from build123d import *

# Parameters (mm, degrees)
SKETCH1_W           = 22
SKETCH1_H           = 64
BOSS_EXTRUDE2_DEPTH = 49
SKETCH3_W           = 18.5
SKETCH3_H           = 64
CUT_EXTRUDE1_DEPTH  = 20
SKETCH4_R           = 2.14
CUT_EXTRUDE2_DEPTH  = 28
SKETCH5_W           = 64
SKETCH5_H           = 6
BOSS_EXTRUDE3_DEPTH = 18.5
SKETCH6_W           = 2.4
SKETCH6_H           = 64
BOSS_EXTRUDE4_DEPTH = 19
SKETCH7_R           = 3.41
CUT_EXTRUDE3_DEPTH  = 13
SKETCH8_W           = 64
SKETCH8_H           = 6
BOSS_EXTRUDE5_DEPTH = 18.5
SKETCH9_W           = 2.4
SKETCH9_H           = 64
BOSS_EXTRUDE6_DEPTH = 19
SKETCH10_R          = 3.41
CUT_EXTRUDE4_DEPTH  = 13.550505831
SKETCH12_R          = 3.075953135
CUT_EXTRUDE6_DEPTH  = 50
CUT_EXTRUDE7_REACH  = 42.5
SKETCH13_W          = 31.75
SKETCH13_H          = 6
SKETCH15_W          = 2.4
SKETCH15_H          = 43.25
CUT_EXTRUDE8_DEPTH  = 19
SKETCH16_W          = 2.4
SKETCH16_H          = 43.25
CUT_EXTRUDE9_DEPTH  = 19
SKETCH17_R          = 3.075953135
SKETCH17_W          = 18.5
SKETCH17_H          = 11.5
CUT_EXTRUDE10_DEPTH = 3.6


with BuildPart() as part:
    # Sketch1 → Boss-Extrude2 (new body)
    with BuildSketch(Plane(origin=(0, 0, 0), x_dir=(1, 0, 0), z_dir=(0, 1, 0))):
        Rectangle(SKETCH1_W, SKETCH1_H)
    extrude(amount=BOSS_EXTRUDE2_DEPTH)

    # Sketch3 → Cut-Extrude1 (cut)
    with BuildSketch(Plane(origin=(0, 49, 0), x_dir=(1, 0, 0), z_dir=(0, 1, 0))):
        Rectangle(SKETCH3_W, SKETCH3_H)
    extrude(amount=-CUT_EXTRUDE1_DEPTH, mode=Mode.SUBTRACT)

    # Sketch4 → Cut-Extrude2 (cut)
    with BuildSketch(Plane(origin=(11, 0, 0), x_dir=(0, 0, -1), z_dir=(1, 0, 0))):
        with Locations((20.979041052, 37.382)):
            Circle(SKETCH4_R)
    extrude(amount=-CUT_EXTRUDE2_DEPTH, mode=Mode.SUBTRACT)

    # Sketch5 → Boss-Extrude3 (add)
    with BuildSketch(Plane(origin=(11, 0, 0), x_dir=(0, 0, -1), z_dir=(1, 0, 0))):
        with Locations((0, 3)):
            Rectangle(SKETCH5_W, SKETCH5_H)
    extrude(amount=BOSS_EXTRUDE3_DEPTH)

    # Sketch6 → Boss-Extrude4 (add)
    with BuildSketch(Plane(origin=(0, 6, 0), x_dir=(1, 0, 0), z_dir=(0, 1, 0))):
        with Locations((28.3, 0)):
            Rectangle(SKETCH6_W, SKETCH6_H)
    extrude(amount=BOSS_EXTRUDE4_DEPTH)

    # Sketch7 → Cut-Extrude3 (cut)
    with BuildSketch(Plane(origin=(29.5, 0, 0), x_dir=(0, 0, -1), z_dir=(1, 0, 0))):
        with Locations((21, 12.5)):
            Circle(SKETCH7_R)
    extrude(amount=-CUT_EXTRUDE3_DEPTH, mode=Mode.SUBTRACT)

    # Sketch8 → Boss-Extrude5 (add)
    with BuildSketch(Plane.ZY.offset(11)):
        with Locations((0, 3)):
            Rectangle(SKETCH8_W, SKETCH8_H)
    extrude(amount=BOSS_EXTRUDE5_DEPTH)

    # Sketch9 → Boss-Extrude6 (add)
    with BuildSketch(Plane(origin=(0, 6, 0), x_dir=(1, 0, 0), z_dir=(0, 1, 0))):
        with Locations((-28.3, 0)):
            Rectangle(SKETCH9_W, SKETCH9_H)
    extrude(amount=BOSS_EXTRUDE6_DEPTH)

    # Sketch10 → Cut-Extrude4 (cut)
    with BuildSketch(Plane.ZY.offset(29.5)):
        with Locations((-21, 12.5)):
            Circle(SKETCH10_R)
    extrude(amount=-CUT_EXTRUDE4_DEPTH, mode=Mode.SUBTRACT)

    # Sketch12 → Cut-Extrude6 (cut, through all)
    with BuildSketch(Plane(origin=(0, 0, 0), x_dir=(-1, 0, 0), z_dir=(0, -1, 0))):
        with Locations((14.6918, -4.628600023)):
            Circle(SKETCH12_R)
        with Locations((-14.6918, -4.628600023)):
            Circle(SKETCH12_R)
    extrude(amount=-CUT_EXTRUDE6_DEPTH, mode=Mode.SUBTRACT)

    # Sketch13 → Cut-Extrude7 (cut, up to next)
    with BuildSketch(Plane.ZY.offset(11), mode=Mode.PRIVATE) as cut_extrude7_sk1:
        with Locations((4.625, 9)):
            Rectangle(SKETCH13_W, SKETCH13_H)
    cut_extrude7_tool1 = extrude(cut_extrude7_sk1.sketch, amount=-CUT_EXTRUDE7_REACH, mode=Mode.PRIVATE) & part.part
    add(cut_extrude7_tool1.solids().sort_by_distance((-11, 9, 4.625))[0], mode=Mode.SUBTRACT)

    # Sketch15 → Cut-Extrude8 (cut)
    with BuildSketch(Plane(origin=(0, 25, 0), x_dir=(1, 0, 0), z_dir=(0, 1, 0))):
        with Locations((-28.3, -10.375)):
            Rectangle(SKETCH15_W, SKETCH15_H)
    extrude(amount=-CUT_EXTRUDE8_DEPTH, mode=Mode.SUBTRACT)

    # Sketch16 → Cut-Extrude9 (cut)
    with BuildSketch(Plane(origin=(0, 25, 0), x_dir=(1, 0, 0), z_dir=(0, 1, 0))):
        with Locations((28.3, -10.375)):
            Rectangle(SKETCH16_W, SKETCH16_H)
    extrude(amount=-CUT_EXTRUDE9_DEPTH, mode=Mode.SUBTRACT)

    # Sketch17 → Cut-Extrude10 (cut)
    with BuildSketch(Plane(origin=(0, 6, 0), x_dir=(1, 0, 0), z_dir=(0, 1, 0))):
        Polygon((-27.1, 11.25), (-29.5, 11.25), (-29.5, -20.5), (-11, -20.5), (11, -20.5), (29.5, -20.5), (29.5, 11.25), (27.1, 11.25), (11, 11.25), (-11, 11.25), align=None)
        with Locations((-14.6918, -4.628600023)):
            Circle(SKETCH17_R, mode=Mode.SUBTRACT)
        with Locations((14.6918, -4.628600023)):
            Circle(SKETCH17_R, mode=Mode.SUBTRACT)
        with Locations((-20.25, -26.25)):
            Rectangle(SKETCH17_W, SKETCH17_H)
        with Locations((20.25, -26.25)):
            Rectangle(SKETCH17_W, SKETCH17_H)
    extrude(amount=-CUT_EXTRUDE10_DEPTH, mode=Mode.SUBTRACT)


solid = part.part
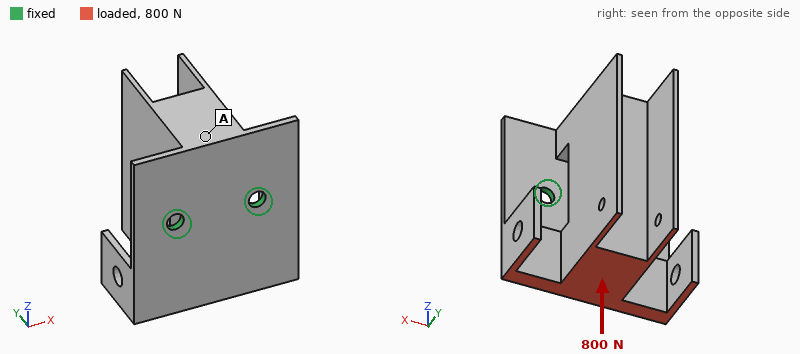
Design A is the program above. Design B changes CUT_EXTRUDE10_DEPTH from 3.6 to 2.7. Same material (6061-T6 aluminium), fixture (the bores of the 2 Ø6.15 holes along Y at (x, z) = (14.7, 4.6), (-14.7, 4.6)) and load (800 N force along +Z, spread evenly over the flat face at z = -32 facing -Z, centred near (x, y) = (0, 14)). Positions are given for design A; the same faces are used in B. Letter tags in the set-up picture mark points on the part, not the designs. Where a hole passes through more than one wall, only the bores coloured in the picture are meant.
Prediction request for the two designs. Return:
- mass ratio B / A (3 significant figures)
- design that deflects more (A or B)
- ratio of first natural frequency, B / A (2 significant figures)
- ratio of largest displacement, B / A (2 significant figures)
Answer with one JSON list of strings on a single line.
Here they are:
["1.04", "A", "1.5", "0.45"]
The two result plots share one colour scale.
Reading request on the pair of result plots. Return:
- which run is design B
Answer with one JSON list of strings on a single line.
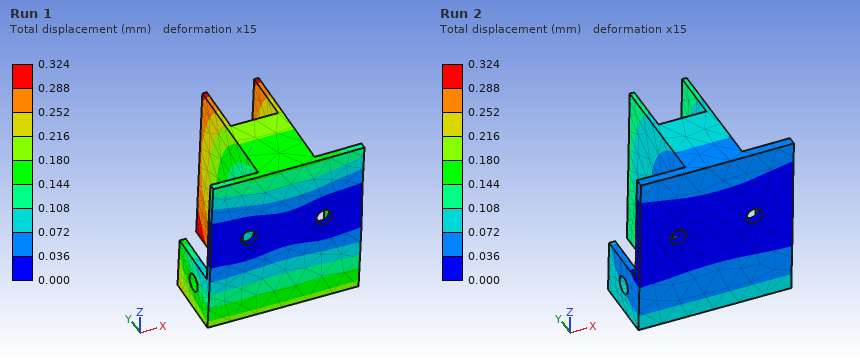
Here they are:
["Run 2"]
